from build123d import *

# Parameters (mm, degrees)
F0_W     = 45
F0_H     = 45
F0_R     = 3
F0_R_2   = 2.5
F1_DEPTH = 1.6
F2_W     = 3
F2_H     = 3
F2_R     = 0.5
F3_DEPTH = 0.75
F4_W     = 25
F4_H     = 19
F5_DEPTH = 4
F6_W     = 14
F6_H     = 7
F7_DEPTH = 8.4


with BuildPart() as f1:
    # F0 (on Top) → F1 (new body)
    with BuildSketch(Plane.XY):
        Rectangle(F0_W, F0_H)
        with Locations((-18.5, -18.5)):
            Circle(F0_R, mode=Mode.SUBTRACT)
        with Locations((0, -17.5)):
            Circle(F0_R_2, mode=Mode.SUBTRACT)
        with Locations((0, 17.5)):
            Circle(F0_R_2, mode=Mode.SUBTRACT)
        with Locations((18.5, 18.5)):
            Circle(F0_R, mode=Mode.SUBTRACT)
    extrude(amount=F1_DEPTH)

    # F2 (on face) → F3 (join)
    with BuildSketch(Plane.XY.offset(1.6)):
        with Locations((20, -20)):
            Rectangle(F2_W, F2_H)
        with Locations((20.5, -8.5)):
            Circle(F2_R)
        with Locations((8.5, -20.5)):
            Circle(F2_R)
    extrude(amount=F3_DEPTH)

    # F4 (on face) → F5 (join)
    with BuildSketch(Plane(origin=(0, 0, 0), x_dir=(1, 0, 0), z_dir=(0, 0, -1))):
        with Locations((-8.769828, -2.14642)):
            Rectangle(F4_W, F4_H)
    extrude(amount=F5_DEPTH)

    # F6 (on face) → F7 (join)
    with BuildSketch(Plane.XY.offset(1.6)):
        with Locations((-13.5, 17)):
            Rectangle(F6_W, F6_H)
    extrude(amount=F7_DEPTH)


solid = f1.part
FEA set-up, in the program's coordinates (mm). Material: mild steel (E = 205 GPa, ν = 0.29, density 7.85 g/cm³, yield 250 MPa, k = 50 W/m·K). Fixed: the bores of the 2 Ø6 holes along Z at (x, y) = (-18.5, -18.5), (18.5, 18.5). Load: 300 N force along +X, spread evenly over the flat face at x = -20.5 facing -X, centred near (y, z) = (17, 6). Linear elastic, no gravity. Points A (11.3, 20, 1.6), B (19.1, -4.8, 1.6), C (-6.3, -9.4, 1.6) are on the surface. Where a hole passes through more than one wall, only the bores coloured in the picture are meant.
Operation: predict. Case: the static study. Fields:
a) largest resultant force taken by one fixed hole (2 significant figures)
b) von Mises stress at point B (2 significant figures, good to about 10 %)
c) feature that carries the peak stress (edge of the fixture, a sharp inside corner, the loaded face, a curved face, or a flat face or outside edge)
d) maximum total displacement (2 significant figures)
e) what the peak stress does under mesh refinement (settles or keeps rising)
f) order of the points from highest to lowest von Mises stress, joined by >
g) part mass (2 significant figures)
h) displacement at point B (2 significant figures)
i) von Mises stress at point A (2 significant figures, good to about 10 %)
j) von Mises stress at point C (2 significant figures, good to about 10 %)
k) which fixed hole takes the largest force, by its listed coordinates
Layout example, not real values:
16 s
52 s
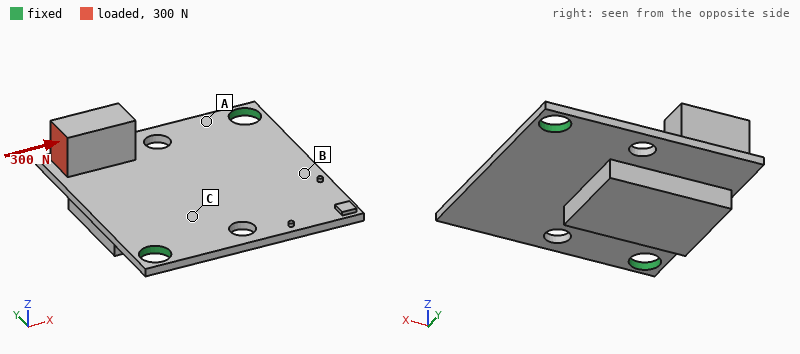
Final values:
260 N
11 MPa
edge of the fixture
76 µm
keeps rising
A > C > B
46 g
35 µm
39 MPa
26 MPa
(18.5, 18.5)
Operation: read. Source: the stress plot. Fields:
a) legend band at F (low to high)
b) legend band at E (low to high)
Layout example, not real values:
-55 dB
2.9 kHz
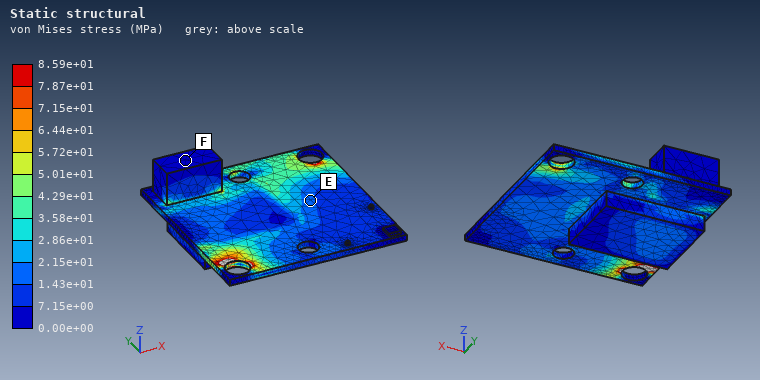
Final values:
0.00e+00 to 7.15e+00 MPa
1.43e+01 to 2.15e+01 MPa
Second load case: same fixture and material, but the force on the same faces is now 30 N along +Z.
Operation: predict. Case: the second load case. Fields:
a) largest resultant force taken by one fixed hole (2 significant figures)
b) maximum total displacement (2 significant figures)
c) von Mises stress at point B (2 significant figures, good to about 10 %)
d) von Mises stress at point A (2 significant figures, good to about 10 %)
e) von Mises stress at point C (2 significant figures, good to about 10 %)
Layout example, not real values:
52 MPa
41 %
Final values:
30 N
57 µm
4.7 MPa
29 MPa
19 MPa
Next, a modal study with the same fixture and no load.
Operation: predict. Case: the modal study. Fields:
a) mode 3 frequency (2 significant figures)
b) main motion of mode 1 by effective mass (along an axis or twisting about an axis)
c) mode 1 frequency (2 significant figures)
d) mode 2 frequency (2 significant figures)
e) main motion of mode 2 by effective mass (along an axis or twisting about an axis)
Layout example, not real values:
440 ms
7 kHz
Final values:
4700 Hz
along Z
1200 Hz
2300 Hz
along Z
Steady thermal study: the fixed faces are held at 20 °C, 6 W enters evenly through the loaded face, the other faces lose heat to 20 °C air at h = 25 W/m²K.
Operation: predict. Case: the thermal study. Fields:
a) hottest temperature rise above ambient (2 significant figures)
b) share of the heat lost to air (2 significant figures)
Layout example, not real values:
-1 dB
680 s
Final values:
55 K
37 %
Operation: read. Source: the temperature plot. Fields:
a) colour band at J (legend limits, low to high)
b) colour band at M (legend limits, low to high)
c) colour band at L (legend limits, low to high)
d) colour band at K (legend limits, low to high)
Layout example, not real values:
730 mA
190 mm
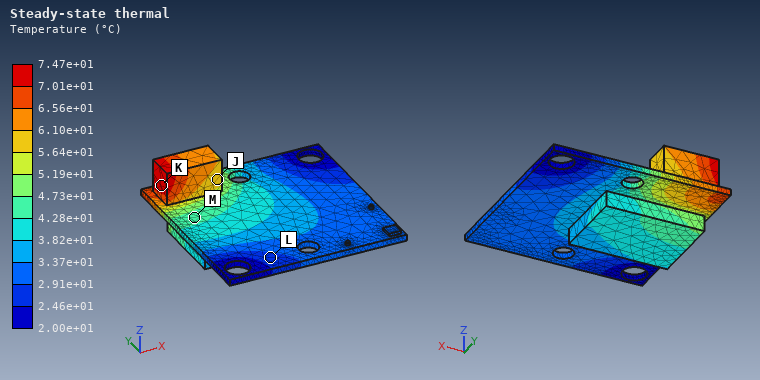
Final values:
5.64e+01 to 6.10e+01 °C
4.28e+01 to 4.73e+01 °C
2.46e+01 to 2.91e+01 °C
7.01e+01 to 7.47e+01 °C
